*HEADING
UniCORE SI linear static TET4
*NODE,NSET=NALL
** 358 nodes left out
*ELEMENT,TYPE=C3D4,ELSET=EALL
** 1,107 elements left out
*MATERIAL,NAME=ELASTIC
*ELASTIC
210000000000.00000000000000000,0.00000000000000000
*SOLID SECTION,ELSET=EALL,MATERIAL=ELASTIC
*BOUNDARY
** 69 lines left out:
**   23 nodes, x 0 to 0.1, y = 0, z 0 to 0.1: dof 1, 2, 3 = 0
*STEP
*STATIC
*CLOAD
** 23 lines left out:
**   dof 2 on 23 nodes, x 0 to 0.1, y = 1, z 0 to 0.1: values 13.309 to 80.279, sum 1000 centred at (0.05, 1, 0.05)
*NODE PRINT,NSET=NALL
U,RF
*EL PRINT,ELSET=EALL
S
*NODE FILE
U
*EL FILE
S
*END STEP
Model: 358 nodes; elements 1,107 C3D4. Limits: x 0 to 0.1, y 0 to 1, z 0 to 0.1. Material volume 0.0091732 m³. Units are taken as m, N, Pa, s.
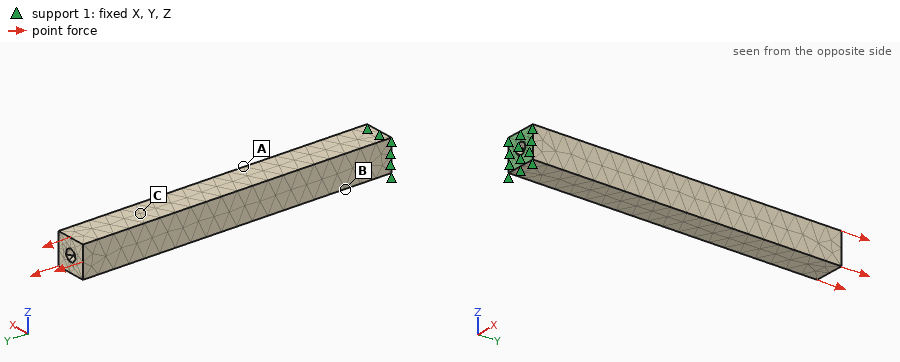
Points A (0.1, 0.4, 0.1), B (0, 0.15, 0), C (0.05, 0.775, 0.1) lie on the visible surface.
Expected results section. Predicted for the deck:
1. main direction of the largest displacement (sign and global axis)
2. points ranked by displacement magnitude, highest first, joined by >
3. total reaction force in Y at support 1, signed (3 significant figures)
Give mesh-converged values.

+Y
C > A > B
-1000 N
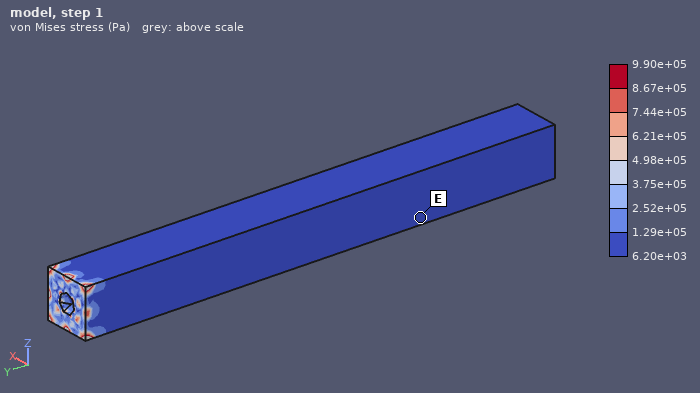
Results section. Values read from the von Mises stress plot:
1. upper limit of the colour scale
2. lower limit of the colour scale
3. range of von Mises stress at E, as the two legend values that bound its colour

9.90e+05 Pa
6.20e+03 Pa
6.20e+03 to 1.29e+05 Pa
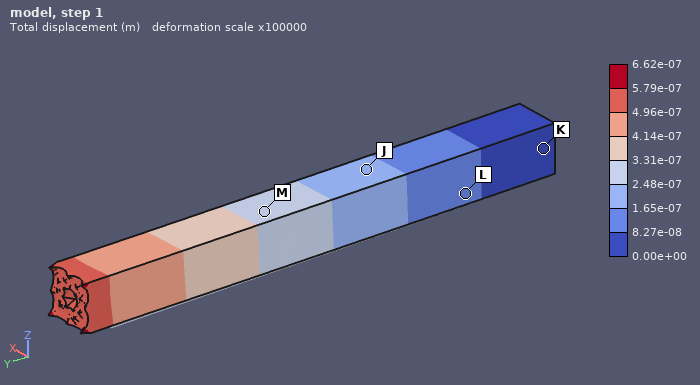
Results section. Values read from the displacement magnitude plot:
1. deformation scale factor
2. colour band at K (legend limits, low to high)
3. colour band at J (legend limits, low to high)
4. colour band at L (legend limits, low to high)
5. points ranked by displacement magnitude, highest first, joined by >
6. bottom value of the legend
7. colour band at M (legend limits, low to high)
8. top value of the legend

100000
0.00e+00 to 8.27e-08 m
1.65e-07 to 2.48e-07 m
8.27e-08 to 1.65e-07 m
M > J > L > K
0.00e+00 m
2.48e-07 to 3.31e-07 m
6.62e-07 m
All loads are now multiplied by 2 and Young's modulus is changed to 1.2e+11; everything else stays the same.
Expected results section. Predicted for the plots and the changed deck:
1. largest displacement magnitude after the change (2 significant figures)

2.3e-06 m
